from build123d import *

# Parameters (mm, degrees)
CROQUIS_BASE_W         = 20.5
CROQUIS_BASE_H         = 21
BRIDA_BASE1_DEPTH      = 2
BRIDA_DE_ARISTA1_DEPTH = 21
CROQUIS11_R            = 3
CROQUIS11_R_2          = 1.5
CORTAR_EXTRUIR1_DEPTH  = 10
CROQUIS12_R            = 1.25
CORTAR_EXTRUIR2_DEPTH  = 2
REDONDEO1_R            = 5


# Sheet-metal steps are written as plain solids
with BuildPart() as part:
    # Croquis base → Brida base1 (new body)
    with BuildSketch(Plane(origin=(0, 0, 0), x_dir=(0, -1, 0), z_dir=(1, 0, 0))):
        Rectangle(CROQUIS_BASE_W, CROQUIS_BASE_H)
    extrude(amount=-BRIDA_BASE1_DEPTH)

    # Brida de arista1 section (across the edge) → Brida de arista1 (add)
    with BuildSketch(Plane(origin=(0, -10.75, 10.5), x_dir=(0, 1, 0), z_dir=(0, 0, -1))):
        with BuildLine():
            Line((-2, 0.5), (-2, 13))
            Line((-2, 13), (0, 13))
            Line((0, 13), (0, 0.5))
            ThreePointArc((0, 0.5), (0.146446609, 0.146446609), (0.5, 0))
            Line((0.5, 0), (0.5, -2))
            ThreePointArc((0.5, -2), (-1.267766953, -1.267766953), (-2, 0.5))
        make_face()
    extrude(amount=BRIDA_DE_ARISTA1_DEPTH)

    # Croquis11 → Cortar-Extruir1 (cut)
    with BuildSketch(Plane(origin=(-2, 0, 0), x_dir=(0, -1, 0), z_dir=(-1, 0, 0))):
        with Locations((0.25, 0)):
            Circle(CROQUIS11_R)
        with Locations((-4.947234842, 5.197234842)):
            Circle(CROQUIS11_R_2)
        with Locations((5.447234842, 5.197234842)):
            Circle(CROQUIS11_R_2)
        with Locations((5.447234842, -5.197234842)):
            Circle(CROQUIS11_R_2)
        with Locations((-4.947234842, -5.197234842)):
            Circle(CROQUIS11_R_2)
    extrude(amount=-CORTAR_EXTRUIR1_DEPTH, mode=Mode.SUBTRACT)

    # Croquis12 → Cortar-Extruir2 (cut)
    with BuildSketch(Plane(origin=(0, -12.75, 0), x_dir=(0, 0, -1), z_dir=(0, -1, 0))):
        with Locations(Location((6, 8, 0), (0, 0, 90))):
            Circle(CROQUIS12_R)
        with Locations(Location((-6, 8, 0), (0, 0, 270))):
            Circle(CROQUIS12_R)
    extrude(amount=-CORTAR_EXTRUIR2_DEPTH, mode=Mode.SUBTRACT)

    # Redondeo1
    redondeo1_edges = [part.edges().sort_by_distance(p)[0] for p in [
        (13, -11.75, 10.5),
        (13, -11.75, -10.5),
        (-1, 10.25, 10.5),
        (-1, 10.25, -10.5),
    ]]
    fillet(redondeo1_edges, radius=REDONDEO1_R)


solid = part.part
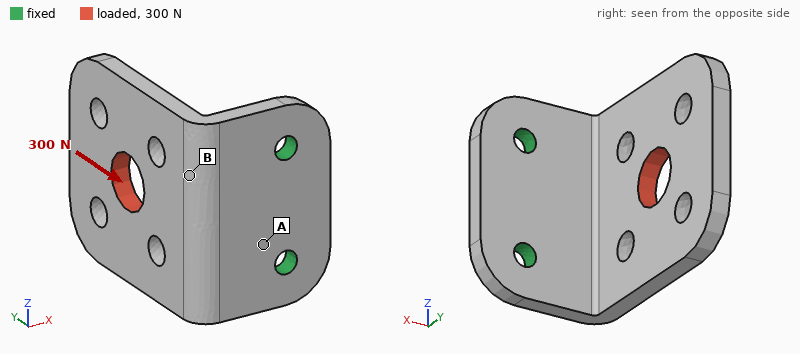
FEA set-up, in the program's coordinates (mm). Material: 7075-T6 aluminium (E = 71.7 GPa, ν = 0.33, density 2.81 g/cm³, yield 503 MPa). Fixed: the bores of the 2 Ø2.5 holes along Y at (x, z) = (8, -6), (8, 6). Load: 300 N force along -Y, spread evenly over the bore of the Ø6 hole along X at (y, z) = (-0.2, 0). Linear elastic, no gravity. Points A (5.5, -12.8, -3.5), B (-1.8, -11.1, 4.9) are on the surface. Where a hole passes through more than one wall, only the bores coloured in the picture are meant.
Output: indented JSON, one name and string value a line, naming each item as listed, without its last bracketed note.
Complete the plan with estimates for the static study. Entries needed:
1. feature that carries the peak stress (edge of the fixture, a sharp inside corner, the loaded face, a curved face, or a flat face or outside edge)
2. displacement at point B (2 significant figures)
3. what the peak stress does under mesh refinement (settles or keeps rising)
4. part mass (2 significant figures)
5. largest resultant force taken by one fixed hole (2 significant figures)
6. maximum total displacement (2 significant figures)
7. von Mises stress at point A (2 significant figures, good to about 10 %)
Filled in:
{
  "feature that carries the peak stress": "edge of the fixture",
  "displacement at point B": "0.076 mm",
  "what the peak stress does under mesh refinement": "keeps rising",
  "part mass": "3.7 g",
  "largest resultant force taken by one fixed hole": "150 N",
  "maximum total displacement": "0.25 mm",
  "von Mises stress at point A": "110 MPa"
}
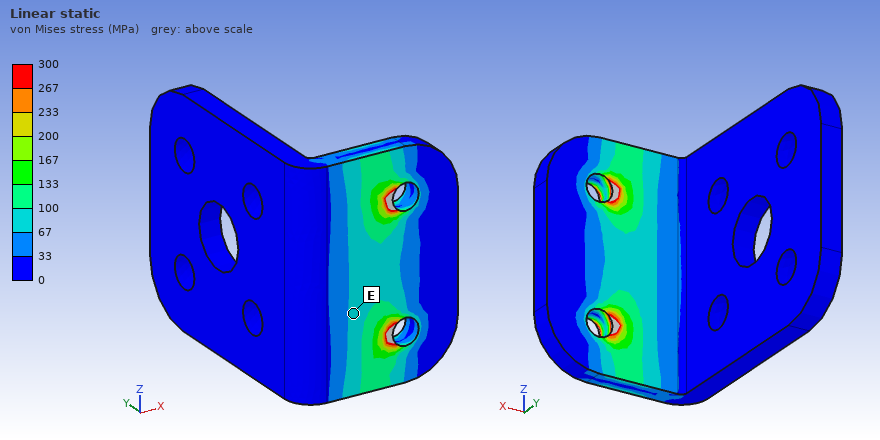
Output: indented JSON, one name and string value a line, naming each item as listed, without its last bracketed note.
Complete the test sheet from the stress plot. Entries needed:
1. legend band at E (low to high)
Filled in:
{
  "legend band at E": "67 to 100 MPa"
}
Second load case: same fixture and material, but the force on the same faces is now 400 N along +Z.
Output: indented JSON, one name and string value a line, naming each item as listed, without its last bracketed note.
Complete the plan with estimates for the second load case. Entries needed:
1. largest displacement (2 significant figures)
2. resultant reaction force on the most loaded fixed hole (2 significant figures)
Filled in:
{
  "largest displacement": "0.24 mm",
  "resultant reaction force on the most loaded fixed hole": "460 N"
}
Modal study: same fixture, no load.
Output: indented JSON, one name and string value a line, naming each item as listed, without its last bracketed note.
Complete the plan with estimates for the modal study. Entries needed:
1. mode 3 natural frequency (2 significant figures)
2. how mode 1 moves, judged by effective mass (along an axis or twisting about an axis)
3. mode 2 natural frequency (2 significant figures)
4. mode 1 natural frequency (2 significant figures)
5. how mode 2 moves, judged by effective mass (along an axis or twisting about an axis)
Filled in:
{
  "mode 3 natural frequency": "8100 Hz",
  "how mode 1 moves, judged by effective mass": "along X",
  "mode 2 natural frequency": "4900 Hz",
  "mode 1 natural frequency": "2300 Hz",
  "how mode 2 moves, judged by effective mass": "along Z"
}
